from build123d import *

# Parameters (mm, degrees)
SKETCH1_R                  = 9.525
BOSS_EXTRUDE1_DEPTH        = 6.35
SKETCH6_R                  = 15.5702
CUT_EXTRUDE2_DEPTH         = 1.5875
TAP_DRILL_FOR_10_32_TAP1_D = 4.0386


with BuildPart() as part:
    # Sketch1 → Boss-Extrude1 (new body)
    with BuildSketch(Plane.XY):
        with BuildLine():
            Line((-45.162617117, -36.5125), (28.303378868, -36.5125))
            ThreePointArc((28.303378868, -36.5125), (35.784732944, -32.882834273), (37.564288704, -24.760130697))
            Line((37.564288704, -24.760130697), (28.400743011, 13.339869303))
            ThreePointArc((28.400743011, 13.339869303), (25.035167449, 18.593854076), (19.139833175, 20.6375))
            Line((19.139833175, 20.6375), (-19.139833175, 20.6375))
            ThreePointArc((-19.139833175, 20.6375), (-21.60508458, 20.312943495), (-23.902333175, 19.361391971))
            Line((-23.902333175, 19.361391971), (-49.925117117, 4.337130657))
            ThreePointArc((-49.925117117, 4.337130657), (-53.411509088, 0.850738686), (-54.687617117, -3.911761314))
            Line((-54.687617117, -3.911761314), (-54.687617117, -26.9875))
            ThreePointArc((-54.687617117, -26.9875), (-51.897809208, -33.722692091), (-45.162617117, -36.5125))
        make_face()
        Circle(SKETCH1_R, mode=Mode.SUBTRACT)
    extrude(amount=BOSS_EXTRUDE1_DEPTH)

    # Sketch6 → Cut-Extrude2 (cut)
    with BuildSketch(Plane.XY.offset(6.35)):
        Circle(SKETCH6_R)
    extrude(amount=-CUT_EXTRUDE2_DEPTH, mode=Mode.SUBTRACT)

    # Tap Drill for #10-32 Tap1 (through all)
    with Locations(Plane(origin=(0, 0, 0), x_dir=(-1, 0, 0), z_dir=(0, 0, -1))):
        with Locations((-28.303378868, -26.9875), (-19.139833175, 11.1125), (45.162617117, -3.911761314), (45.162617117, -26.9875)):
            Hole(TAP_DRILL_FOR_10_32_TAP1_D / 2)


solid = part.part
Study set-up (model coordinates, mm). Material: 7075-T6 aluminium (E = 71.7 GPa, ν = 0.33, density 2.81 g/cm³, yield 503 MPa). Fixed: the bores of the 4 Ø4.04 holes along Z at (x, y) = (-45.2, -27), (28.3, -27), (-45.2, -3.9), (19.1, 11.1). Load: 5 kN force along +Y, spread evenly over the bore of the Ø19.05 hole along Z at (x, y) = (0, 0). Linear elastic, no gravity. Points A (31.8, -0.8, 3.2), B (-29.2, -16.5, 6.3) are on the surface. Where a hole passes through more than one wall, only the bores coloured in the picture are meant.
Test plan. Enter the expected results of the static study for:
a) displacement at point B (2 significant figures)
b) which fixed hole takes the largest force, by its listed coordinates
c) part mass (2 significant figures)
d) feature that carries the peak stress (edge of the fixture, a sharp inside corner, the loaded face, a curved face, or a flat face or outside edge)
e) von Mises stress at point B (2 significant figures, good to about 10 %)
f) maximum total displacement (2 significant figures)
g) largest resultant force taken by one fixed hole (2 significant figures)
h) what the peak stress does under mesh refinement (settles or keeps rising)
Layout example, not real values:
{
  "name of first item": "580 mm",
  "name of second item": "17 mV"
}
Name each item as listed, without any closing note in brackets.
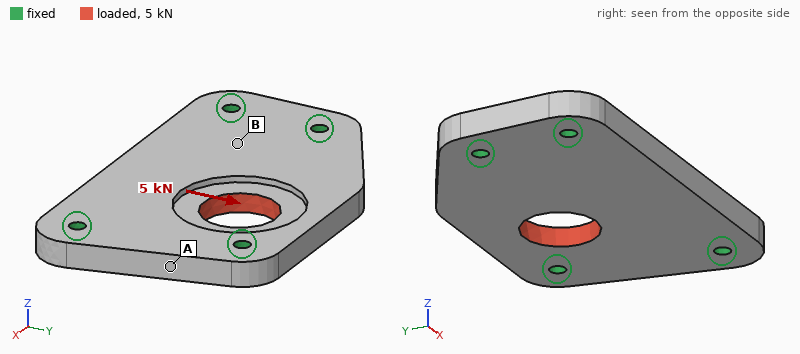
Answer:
{
  "displacement at point B": "5.4 µm",
  "which fixed hole takes the largest force, by its listed coordinates": "(19.1, 11.1)",
  "part mass": "75 g",
  "feature that carries the peak stress": "edge of the fixture",
  "von Mises stress at point B": "13 MPa",
  "maximum total displacement": "17 µm",
  "largest resultant force taken by one fixed hole": "2.2 kN",
  "what the peak stress does under mesh refinement": "keeps rising"
}
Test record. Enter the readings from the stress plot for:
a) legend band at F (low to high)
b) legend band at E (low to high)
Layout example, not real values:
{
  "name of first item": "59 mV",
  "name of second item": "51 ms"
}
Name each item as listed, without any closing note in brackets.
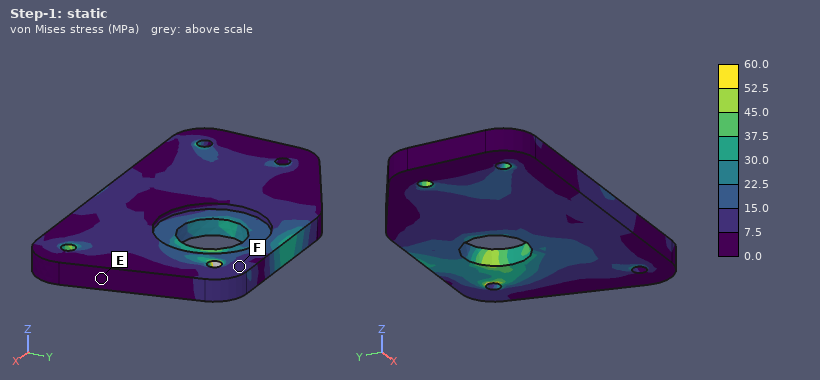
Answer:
{
  "legend band at F": "7.5 to 15.0 MPa",
  "legend band at E": "0.0 to 7.5 MPa"
}
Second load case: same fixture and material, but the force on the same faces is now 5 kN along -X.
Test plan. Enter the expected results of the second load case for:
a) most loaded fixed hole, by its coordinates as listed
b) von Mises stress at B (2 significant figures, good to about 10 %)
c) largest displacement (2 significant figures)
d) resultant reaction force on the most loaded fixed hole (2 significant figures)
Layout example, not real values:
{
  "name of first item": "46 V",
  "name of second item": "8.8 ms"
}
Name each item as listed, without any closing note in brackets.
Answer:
{
  "most loaded fixed hole, by its coordinates as listed": "(19.1, 11.1)",
  "von Mises stress at B": "6.0 MPa",
  "largest displacement": "7.6 µm",
  "resultant reaction force on the most loaded fixed hole": "2.1 kN"
}
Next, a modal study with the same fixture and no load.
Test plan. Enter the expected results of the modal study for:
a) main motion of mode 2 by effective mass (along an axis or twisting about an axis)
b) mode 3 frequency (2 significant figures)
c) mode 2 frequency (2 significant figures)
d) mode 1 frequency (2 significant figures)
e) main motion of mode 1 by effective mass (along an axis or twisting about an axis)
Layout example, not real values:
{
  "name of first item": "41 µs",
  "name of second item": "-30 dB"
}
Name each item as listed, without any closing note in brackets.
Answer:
{
  "main motion of mode 2 by effective mass": "twisting about X",
  "mode 3 frequency": "13 kHz",
  "mode 2 frequency": "6700 Hz",
  "mode 1 frequency": "5800 Hz",
  "main motion of mode 1 by effective mass": "along Z"
}
